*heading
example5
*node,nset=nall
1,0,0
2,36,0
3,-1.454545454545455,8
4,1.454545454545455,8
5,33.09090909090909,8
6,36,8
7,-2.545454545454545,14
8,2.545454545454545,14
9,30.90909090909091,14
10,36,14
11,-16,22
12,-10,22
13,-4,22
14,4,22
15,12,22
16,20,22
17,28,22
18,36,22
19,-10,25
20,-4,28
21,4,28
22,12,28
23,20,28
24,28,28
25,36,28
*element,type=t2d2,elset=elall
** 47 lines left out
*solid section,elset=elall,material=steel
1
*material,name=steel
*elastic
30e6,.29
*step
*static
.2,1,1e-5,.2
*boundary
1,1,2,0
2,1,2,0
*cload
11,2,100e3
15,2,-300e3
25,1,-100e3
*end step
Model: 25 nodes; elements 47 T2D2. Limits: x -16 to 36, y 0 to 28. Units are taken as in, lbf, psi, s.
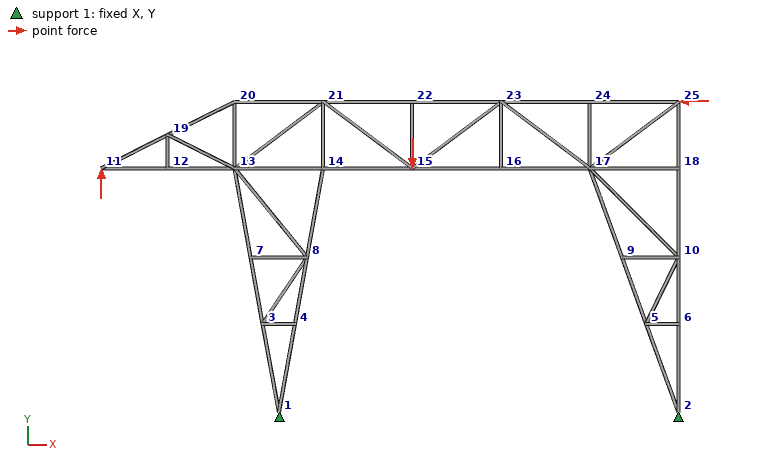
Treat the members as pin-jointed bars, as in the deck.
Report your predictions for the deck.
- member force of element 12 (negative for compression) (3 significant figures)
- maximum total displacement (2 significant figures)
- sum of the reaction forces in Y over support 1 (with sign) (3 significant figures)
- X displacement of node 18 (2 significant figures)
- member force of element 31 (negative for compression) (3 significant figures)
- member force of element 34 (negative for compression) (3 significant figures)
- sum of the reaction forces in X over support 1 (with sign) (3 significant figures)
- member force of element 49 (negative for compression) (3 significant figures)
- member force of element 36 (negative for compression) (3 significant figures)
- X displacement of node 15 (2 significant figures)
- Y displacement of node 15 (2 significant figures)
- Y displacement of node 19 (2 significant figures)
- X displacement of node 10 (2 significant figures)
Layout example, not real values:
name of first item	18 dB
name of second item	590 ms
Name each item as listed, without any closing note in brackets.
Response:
member force of element 12 (negative for compression)	-59300 lbf
maximum total displacement	1.4 in
sum of the reaction forces in Y over support 1 (with sign)	2.00e+05 lbf
X displacement of node 18	-0.97 in
member force of element 31 (negative for compression)	-3.49e+05 lbf
member force of element 34 (negative for compression)	-3.57e+05 lbf
sum of the reaction forces in X over support 1 (with sign)	1.00e+05 lbf
member force of element 49 (negative for compression)	98900 lbf
member force of element 36 (negative for compression)	3.89e+05 lbf
X displacement of node 15	-1.1 in
Y displacement of node 15	-0.61 in
Y displacement of node 19	0.27 in
X displacement of node 10	-0.64 in
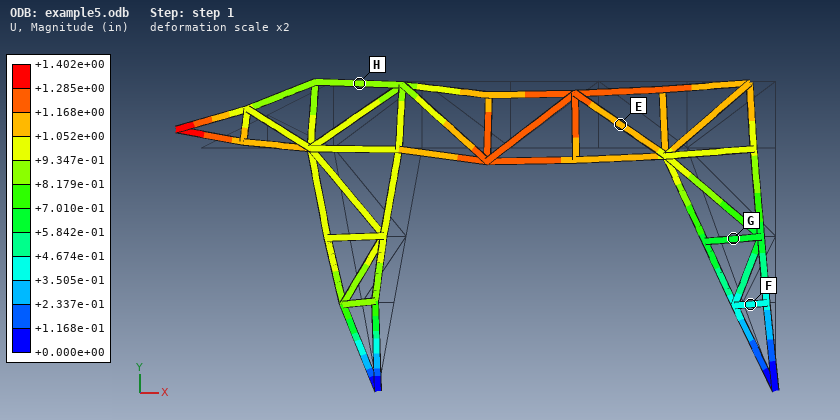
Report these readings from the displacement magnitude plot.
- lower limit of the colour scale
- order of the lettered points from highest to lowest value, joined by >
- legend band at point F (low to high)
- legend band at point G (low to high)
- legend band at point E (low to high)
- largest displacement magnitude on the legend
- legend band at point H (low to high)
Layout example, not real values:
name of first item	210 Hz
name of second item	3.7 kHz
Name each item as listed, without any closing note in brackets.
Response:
lower limit of the colour scale	+0.000e+00 in
order of the lettered points from highest to lowest value, joined by >	E > H > G > F
legend band at point F	+3.505e-01 to +4.674e-01 in
legend band at point G	+5.842e-01 to +7.010e-01 in
legend band at point E	+1.052e+00 to +1.168e+00 in
largest displacement magnitude on the legend	+1.402e+00 in
legend band at point H	+8.179e-01 to +9.347e-01 in
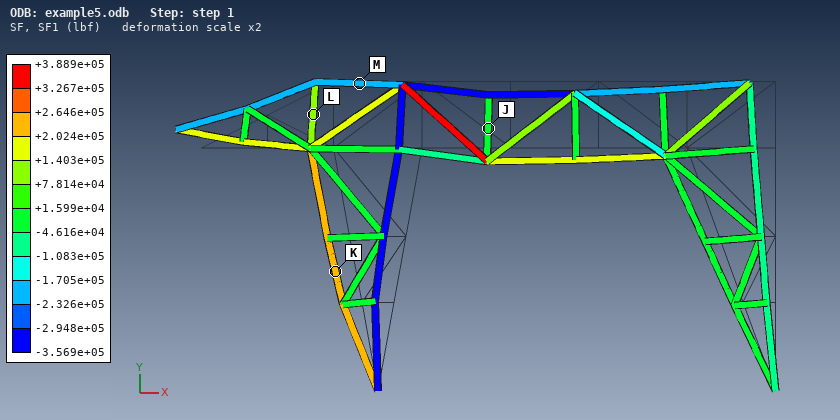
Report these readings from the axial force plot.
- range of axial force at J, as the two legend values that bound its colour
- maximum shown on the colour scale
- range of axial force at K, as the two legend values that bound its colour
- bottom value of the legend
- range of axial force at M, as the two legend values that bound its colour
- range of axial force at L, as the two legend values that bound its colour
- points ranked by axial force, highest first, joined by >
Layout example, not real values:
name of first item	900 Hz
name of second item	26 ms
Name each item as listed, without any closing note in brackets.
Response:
range of axial force at J, as the two legend values that bound its colour	-4.616e+04 to +1.599e+04 lbf
maximum shown on the colour scale	+3.889e+05 lbf
range of axial force at K, as the two legend values that bound its colour	+2.024e+05 to +2.646e+05 lbf
bottom value of the legend	-3.569e+05 lbf
range of axial force at M, as the two legend values that bound its colour	-2.326e+05 to -1.705e+05 lbf
range of axial force at L, as the two legend values that bound its colour	+7.814e+04 to +1.403e+05 lbf
points ranked by axial force, highest first, joined by >	K > L > J > M
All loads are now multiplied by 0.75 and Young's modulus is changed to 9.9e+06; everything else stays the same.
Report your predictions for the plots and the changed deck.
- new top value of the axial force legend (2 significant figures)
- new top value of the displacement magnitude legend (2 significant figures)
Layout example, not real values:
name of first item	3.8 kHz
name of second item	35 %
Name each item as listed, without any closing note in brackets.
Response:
new top value of the axial force legend	2.9e+05 lbf
new top value of the displacement magnitude legend	3.2 in
